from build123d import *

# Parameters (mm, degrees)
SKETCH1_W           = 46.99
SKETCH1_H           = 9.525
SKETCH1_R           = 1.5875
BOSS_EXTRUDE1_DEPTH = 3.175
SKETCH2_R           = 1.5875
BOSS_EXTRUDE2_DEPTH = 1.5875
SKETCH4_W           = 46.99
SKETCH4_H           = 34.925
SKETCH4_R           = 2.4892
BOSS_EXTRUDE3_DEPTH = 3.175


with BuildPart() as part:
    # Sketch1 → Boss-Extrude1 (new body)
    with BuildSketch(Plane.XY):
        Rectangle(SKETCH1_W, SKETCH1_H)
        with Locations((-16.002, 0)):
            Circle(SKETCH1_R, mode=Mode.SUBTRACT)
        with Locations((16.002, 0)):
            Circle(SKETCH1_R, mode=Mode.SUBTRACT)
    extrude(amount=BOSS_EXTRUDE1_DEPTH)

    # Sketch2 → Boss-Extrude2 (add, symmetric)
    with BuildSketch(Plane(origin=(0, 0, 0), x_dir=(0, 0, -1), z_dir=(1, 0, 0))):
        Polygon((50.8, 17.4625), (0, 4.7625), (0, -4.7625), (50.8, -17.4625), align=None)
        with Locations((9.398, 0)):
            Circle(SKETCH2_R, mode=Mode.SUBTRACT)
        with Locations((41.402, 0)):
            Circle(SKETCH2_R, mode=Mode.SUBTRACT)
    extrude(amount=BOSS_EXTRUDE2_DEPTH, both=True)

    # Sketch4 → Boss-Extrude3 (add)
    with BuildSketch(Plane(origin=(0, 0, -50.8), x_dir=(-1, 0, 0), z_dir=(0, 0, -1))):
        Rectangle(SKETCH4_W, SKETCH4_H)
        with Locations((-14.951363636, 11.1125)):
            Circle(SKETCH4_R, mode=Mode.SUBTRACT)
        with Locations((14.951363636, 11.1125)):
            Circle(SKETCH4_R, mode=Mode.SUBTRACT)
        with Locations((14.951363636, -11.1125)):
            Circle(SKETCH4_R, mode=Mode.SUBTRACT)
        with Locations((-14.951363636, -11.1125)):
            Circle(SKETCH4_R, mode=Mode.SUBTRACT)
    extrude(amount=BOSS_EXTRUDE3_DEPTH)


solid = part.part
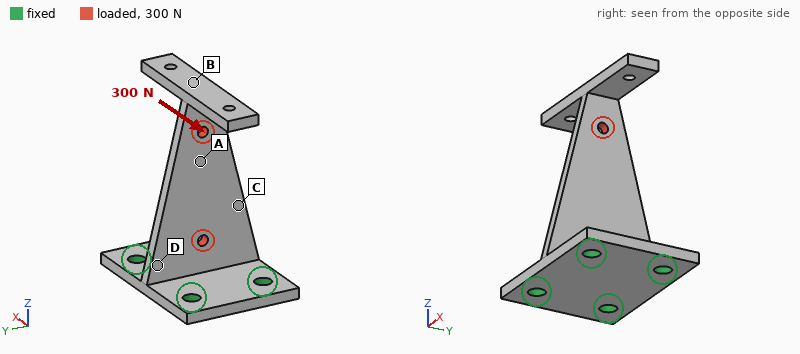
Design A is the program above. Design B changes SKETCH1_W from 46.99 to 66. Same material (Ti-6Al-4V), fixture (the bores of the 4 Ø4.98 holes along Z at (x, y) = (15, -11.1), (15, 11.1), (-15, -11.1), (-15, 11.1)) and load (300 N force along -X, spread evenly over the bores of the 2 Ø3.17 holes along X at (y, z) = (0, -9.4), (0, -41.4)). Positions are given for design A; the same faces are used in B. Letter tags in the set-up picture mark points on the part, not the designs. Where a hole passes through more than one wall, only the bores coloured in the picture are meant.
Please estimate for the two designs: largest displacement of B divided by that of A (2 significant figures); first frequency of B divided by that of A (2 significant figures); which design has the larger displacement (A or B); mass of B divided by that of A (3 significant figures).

1.1
0.81
B
1.06
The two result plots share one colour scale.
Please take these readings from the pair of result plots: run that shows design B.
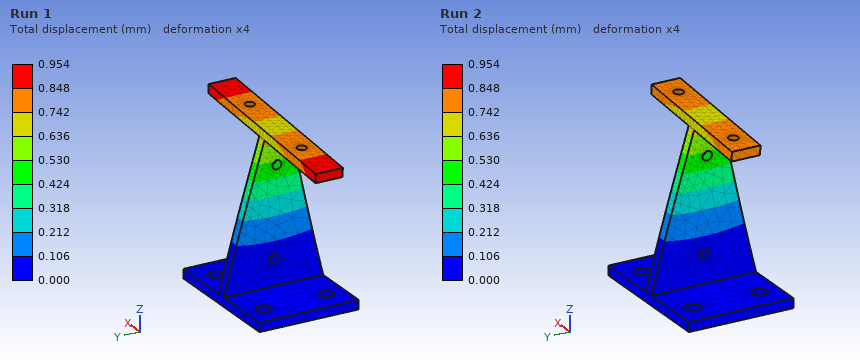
Run 1
